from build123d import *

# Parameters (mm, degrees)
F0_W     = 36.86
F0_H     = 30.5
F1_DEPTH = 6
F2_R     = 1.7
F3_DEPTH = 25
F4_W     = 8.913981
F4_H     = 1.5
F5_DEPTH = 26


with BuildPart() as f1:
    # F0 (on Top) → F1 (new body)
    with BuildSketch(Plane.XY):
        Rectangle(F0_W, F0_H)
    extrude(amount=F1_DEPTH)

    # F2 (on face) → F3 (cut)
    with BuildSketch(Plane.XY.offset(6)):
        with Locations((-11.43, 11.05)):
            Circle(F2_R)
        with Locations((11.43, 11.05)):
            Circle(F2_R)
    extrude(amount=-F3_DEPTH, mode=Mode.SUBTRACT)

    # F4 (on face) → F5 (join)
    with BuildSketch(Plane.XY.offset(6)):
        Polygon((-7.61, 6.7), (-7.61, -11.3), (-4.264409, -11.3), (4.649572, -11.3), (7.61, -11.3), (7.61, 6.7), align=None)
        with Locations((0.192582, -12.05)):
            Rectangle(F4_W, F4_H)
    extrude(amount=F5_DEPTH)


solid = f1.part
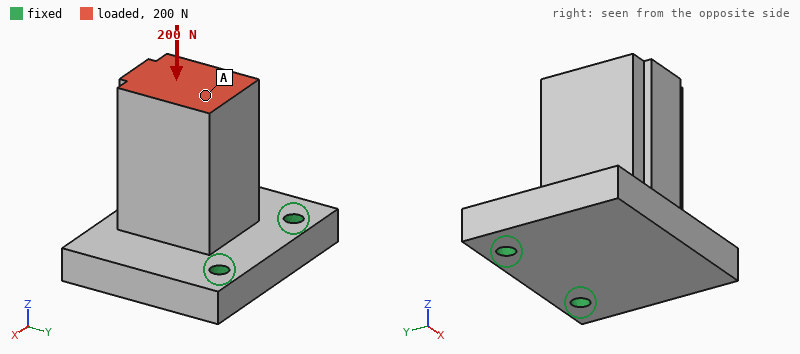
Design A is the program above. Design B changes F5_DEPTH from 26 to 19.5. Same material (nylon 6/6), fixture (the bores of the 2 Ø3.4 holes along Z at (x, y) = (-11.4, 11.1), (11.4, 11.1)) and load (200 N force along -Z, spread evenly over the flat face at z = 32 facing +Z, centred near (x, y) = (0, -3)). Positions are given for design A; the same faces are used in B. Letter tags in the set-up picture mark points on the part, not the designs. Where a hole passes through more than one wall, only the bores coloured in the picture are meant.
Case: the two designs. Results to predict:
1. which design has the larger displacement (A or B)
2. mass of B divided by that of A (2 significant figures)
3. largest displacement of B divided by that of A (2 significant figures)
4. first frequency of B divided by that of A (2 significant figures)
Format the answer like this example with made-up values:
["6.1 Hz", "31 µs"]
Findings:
["A", "0.87", "0.87", "1.2"]
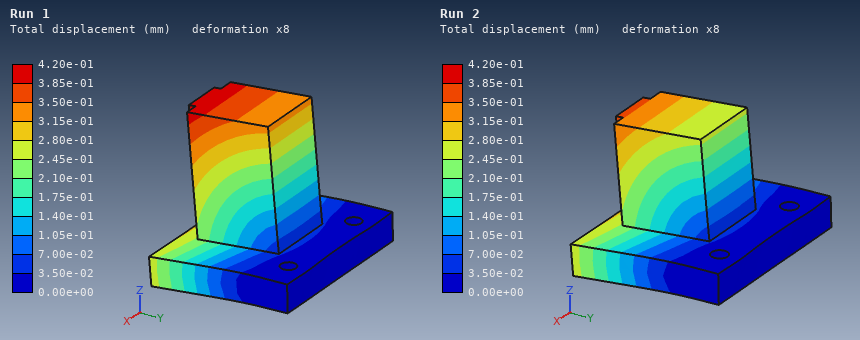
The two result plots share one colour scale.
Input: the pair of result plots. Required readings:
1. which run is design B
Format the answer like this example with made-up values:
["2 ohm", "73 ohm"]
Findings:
["Run 2"]
